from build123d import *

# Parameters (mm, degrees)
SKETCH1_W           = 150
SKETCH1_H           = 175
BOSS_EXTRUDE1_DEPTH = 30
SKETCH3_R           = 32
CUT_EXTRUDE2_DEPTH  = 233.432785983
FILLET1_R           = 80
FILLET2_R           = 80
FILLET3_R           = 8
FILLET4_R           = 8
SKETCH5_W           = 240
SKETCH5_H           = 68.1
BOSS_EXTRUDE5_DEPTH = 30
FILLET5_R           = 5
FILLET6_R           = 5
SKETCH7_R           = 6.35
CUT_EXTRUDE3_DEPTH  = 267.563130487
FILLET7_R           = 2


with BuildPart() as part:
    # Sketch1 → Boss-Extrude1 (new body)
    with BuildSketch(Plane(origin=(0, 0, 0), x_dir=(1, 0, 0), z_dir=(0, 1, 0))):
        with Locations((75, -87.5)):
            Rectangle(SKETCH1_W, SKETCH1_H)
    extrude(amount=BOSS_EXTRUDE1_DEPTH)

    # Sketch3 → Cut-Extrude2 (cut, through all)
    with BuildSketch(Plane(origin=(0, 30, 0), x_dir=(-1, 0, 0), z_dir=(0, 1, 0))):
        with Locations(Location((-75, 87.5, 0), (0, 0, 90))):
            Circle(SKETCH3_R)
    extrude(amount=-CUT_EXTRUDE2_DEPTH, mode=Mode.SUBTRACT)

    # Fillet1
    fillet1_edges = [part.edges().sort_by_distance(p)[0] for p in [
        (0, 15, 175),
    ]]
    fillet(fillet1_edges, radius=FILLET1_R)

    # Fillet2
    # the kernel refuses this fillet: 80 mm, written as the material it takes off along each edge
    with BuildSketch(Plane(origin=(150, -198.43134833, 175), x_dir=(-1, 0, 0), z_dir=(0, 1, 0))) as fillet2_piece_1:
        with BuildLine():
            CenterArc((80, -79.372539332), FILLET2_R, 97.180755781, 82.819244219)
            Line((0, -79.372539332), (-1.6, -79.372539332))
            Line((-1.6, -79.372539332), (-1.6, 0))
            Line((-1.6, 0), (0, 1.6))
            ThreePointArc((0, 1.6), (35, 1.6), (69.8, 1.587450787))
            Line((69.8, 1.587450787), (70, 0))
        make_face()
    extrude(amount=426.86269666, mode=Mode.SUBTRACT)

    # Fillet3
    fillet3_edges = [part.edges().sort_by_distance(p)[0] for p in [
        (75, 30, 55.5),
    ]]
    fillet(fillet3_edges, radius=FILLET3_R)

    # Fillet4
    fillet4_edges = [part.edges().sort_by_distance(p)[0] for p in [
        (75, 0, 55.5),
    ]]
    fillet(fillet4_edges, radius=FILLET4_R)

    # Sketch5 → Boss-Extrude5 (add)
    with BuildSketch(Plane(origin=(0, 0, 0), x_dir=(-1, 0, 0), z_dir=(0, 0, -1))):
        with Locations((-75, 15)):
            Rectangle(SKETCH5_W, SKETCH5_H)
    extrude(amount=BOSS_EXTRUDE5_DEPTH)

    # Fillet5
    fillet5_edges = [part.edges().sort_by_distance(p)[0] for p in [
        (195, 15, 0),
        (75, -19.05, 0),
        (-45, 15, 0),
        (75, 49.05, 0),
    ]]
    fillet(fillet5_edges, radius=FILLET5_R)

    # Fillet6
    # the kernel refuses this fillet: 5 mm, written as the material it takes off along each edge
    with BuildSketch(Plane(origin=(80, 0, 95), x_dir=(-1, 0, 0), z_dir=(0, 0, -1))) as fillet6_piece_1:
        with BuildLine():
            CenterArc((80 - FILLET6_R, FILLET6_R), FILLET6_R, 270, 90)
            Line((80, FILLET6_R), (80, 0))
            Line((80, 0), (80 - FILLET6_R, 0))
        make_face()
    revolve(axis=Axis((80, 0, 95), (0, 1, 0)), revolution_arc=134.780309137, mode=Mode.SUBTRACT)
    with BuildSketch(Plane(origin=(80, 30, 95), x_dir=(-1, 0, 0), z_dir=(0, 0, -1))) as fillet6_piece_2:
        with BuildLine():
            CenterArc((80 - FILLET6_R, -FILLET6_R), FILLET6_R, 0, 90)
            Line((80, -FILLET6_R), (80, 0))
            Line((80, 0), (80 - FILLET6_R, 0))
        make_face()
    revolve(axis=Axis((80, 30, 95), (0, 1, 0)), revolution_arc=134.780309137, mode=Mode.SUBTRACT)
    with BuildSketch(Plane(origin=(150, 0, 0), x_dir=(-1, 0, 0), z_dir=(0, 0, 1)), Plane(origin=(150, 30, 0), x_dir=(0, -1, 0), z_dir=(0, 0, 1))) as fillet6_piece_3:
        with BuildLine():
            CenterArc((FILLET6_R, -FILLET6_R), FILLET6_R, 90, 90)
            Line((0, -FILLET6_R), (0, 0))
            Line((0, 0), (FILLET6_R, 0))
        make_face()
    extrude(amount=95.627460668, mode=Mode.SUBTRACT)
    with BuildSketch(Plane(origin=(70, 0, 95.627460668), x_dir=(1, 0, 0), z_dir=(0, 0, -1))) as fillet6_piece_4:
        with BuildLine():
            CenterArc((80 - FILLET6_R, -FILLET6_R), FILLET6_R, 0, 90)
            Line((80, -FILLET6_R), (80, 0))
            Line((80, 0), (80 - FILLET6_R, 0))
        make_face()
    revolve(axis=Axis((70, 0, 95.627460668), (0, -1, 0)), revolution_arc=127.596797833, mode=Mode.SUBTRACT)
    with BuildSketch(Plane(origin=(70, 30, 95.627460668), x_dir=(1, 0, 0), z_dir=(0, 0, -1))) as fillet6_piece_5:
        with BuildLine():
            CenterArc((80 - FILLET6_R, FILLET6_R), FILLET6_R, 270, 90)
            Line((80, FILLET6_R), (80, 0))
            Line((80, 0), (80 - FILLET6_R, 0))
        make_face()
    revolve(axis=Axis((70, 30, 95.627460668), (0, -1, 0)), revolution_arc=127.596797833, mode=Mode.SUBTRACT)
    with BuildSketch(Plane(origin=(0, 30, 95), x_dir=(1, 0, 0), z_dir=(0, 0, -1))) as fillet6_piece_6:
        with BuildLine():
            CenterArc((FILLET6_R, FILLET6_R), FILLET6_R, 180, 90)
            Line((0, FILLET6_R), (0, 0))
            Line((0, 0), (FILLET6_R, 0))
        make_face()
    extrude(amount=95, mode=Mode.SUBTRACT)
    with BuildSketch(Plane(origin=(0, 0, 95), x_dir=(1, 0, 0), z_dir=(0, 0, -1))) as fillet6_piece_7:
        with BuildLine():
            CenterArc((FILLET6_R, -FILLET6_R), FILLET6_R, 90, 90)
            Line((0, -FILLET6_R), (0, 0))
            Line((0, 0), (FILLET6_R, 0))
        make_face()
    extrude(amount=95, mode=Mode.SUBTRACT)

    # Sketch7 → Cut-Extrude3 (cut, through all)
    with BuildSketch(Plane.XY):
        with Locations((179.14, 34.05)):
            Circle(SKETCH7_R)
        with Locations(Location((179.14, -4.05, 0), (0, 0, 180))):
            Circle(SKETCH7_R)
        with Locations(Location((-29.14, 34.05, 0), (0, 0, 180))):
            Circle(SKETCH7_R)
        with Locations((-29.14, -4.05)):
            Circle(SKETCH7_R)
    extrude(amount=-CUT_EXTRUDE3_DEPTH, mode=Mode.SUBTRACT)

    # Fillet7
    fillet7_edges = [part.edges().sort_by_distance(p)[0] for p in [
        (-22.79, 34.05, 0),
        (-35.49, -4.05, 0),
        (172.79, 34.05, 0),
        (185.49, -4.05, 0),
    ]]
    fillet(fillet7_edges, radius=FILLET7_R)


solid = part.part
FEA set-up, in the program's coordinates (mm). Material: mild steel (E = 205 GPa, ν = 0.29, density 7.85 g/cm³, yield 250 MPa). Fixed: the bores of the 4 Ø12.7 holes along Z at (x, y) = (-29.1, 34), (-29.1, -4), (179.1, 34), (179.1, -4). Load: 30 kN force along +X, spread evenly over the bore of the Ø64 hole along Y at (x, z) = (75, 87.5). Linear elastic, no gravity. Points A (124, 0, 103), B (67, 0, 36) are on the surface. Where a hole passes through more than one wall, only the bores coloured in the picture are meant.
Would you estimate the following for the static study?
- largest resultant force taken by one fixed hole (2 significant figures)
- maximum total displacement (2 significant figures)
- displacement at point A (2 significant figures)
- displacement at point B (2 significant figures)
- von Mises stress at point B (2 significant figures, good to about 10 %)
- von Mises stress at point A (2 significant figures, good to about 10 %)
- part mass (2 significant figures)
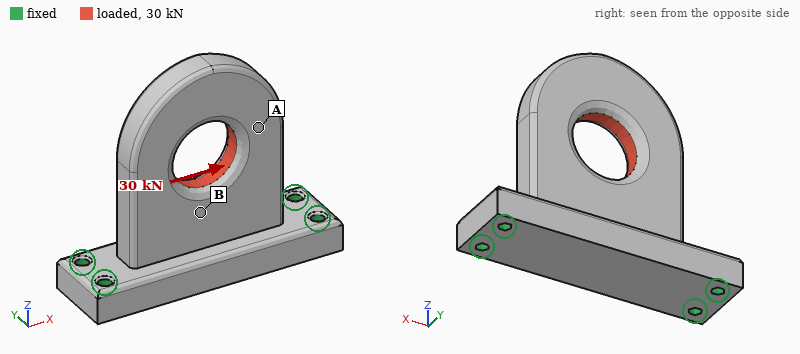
12 kN
51 µm
37 µm
12 µm
21 MPa
9.7 MPa
8.4 kg
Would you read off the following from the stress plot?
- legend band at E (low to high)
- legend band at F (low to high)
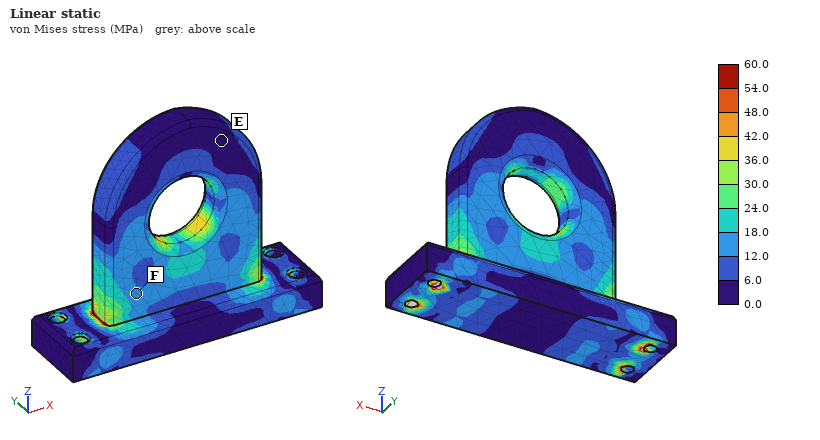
0.0 to 6.0 MPa
12.0 to 18.0 MPa
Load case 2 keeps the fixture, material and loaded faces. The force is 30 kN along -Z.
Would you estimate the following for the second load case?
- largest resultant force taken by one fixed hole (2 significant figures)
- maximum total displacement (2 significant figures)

8.1 kN
16 µm
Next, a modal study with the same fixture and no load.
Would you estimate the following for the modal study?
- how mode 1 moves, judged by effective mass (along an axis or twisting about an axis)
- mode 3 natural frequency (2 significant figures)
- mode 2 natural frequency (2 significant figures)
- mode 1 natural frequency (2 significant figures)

along Y
2100 Hz
2100 Hz
650 Hz
